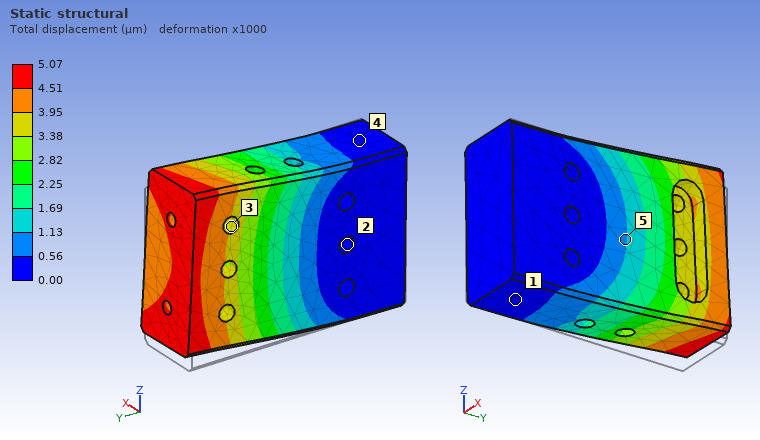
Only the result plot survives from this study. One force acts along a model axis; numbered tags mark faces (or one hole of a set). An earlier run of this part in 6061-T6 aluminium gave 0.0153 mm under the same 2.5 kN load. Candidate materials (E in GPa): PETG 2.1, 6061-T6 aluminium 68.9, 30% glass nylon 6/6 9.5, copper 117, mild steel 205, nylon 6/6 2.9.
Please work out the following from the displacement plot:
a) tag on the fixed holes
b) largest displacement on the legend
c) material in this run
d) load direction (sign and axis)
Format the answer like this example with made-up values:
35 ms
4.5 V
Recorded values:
2
5.07 µm
mild steel
+Z
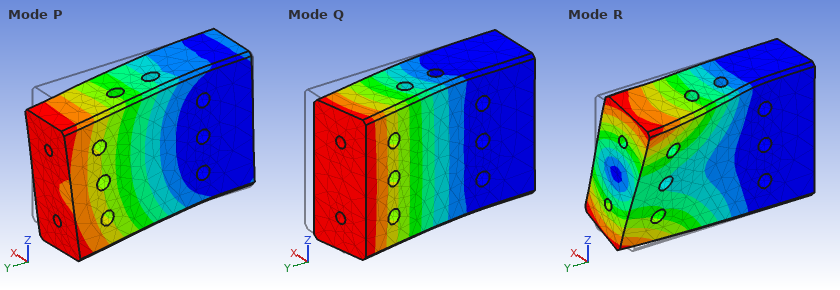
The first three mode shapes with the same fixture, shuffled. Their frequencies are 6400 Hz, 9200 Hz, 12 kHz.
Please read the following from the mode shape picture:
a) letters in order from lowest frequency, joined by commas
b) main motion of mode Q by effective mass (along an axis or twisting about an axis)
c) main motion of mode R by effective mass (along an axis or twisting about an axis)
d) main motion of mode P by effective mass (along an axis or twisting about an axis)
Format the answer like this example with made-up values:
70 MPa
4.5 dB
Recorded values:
Q, P, R
along X
twisting about Y
along Z
